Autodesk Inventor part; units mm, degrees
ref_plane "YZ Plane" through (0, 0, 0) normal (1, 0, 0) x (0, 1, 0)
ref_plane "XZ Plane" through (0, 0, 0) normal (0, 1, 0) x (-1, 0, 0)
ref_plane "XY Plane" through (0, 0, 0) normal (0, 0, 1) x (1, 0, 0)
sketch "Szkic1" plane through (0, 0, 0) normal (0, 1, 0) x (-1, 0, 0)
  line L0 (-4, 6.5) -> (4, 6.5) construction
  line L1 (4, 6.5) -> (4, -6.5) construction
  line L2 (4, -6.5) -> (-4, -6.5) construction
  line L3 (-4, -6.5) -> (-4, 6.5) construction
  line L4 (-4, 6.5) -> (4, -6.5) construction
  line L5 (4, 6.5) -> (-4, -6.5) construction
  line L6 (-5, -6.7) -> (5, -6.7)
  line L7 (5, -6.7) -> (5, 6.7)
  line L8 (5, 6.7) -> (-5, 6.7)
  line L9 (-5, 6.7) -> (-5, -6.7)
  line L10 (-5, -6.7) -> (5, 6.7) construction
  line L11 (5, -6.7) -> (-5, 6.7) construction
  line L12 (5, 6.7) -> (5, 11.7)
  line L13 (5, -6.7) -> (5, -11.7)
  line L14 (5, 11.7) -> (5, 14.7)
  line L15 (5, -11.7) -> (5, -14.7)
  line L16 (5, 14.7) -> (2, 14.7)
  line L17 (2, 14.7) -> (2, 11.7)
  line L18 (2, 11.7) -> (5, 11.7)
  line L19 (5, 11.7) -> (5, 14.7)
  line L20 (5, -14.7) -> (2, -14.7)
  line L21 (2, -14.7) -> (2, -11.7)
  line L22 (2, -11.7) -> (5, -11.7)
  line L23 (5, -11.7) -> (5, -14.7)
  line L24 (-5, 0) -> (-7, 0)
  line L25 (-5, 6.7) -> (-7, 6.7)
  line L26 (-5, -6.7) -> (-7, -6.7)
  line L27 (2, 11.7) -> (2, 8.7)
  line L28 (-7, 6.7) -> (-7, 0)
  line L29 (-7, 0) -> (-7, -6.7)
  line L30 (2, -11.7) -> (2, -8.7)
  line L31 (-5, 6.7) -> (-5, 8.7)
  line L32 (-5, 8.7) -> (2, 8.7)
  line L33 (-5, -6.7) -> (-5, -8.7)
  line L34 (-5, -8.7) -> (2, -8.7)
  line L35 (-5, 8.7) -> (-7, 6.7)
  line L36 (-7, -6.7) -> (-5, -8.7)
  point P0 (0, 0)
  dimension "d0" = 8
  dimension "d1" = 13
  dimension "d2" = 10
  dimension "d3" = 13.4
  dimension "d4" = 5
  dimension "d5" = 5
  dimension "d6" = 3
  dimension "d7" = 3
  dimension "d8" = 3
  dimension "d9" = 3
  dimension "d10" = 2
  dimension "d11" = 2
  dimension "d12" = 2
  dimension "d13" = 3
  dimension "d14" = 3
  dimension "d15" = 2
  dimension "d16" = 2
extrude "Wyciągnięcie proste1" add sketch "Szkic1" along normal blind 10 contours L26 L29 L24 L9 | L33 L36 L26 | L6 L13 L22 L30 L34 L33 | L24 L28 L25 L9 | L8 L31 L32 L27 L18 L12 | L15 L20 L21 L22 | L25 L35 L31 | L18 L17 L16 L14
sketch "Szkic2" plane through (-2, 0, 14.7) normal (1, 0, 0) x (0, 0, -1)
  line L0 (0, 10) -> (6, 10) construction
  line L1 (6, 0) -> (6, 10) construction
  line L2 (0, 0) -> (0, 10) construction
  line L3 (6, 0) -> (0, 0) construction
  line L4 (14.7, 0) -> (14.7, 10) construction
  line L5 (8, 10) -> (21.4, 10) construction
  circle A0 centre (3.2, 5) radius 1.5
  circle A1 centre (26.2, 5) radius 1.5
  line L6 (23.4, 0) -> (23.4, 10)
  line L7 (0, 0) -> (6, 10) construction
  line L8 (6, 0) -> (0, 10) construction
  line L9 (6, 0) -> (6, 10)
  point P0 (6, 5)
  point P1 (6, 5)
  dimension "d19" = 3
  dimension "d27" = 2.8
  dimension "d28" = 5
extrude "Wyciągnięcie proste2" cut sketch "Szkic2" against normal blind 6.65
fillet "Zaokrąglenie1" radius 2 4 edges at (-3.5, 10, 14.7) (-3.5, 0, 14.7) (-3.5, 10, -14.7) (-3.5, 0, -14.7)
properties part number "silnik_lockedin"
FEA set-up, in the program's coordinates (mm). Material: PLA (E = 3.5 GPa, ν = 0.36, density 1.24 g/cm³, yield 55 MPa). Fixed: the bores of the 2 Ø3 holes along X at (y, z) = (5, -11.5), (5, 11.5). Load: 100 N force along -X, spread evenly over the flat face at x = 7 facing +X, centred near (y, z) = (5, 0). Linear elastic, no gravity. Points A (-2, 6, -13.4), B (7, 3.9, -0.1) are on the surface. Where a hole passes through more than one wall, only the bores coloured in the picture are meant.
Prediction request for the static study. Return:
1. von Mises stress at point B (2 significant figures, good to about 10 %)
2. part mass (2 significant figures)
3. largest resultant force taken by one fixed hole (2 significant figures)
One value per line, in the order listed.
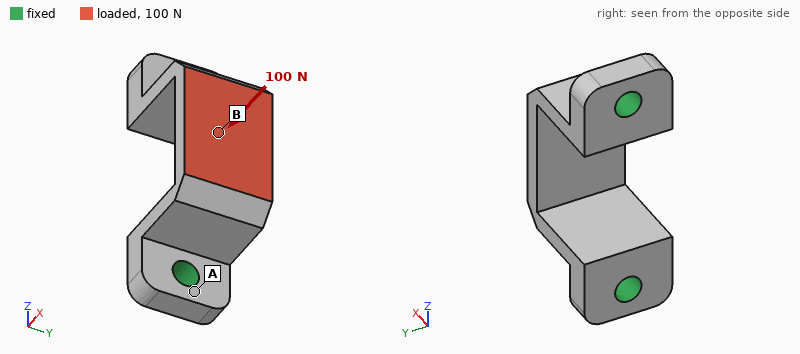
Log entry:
15 MPa
1.3 g
54 N
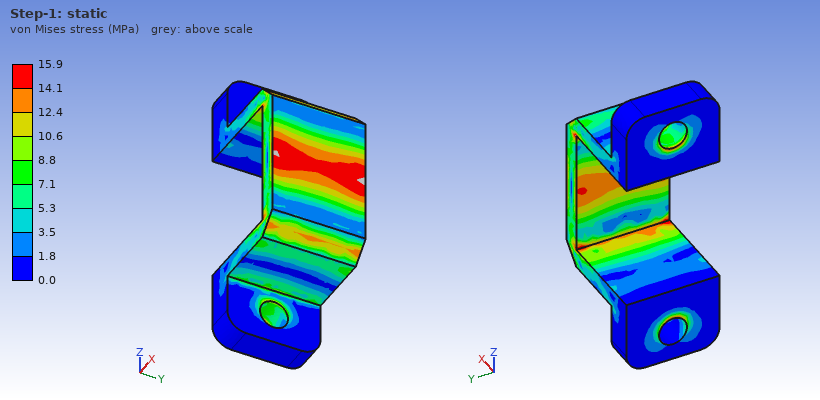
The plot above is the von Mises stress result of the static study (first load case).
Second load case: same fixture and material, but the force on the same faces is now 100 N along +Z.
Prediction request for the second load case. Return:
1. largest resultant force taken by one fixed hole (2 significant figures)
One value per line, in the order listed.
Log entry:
59 N
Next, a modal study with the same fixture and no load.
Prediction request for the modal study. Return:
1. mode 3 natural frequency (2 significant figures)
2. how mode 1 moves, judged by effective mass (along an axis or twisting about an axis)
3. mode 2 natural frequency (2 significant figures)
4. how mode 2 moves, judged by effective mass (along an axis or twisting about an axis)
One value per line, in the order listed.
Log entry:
7700 Hz
along Z
5300 Hz
along Y
